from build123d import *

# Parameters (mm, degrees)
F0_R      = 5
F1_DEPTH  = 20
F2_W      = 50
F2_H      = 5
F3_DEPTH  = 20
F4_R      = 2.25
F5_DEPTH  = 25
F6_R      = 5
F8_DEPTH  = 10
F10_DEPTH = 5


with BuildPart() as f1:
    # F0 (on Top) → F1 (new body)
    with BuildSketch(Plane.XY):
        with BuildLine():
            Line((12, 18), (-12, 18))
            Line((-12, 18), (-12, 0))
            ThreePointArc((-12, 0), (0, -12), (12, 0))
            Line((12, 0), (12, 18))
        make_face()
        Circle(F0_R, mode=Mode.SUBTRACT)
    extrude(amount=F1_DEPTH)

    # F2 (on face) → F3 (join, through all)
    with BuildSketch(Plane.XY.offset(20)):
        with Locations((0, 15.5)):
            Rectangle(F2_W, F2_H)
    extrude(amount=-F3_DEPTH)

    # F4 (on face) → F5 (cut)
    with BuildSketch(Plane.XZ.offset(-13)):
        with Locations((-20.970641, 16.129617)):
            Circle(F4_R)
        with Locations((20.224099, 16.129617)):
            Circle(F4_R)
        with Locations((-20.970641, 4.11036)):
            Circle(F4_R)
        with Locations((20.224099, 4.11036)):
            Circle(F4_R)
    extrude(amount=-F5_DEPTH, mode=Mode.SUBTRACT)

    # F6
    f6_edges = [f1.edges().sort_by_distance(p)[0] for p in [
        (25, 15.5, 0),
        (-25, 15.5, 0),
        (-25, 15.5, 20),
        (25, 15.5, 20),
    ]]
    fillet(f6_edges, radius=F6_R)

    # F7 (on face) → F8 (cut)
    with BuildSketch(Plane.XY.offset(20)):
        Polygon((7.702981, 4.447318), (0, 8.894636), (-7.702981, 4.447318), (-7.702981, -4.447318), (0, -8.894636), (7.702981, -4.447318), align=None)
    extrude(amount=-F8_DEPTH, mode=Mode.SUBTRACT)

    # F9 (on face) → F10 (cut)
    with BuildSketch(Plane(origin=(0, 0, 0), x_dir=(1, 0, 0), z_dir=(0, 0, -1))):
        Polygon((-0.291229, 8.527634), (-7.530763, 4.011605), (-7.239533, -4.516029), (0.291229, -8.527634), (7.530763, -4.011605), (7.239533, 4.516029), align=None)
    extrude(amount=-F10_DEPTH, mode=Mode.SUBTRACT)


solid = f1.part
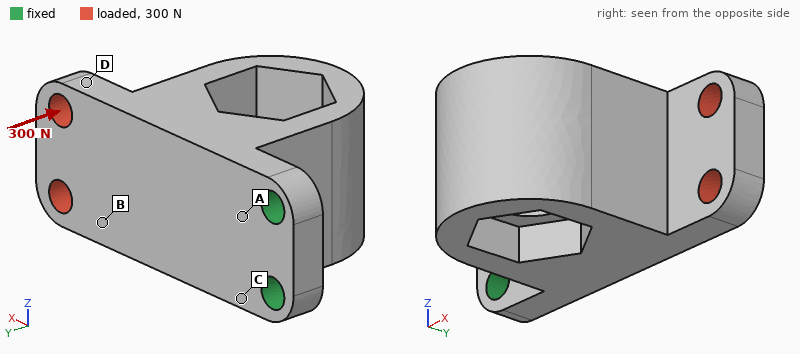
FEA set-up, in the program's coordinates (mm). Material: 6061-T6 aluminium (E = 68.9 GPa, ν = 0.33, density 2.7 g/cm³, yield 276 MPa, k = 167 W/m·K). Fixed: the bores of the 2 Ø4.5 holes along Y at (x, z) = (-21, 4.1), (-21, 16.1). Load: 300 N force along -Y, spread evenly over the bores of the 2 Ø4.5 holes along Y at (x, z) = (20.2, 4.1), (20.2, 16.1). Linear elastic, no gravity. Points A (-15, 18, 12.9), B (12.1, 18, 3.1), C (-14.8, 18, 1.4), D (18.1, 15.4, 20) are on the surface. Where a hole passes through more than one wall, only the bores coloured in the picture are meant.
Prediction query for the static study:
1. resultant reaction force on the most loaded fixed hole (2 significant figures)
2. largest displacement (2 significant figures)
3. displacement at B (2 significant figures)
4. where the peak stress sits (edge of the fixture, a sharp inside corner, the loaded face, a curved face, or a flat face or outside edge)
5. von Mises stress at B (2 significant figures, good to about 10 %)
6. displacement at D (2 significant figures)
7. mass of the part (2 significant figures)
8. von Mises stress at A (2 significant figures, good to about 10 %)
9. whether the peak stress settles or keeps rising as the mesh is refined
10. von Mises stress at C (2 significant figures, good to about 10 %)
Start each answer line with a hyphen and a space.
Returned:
- 150 N
- 0.32 mm
- 0.21 mm
- edge of the fixture
- 24 MPa
- 0.26 mm
- 32 g
- 110 MPa
- keeps rising
- 130 MPa
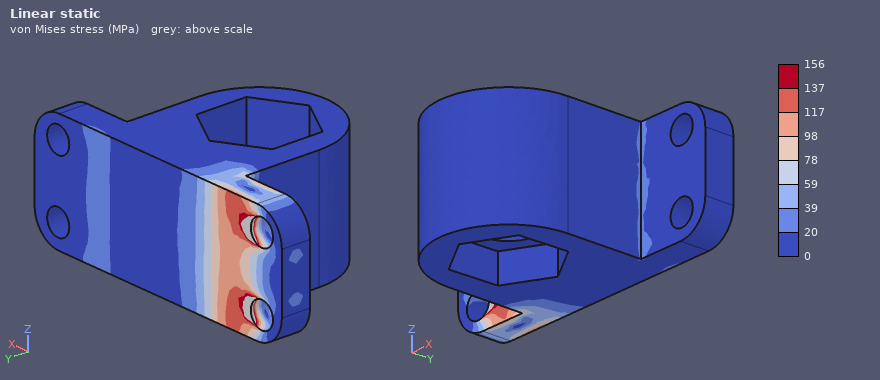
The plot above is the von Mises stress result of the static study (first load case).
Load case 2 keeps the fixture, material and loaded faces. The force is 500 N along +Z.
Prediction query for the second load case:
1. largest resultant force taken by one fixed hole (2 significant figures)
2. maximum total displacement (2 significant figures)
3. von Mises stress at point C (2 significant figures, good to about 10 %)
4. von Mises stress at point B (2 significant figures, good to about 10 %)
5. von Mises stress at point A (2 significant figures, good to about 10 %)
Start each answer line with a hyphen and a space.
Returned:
- 1.5 kN
- 58 µm
- 35 MPa
- 8.5 MPa
- 23 MPa
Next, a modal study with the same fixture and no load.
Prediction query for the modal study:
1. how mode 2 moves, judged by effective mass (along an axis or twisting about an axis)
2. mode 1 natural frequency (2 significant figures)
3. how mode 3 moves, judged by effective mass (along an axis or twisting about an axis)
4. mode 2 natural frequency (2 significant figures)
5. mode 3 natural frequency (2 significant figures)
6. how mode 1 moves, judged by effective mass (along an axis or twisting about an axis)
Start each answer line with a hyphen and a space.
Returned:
- along Z
- 1500 Hz
- along Z
- 4100 Hz
- 6700 Hz
- along Y
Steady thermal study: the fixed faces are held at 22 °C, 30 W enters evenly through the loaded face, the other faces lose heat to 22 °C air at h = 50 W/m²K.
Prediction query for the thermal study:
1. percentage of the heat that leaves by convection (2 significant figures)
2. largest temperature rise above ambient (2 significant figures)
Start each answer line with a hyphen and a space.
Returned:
- 18 %
- 52 K
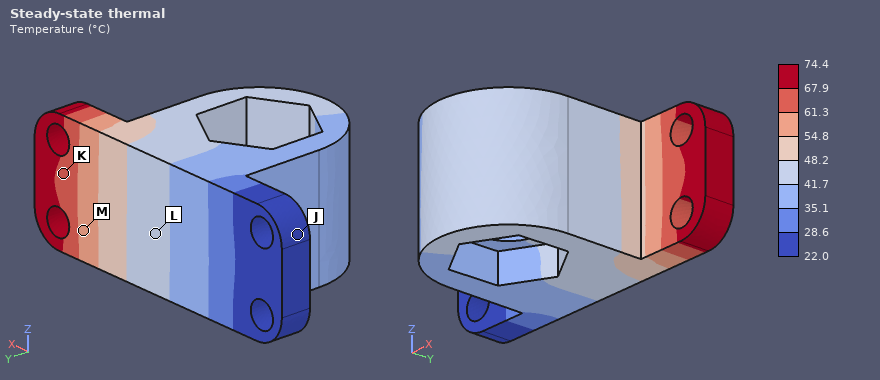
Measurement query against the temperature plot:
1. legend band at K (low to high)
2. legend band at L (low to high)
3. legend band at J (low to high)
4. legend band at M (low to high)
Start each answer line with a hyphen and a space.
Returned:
- 61.3 to 67.9 °C
- 41.7 to 48.2 °C
- 22.0 to 28.6 °C
- 54.8 to 61.3 °C
